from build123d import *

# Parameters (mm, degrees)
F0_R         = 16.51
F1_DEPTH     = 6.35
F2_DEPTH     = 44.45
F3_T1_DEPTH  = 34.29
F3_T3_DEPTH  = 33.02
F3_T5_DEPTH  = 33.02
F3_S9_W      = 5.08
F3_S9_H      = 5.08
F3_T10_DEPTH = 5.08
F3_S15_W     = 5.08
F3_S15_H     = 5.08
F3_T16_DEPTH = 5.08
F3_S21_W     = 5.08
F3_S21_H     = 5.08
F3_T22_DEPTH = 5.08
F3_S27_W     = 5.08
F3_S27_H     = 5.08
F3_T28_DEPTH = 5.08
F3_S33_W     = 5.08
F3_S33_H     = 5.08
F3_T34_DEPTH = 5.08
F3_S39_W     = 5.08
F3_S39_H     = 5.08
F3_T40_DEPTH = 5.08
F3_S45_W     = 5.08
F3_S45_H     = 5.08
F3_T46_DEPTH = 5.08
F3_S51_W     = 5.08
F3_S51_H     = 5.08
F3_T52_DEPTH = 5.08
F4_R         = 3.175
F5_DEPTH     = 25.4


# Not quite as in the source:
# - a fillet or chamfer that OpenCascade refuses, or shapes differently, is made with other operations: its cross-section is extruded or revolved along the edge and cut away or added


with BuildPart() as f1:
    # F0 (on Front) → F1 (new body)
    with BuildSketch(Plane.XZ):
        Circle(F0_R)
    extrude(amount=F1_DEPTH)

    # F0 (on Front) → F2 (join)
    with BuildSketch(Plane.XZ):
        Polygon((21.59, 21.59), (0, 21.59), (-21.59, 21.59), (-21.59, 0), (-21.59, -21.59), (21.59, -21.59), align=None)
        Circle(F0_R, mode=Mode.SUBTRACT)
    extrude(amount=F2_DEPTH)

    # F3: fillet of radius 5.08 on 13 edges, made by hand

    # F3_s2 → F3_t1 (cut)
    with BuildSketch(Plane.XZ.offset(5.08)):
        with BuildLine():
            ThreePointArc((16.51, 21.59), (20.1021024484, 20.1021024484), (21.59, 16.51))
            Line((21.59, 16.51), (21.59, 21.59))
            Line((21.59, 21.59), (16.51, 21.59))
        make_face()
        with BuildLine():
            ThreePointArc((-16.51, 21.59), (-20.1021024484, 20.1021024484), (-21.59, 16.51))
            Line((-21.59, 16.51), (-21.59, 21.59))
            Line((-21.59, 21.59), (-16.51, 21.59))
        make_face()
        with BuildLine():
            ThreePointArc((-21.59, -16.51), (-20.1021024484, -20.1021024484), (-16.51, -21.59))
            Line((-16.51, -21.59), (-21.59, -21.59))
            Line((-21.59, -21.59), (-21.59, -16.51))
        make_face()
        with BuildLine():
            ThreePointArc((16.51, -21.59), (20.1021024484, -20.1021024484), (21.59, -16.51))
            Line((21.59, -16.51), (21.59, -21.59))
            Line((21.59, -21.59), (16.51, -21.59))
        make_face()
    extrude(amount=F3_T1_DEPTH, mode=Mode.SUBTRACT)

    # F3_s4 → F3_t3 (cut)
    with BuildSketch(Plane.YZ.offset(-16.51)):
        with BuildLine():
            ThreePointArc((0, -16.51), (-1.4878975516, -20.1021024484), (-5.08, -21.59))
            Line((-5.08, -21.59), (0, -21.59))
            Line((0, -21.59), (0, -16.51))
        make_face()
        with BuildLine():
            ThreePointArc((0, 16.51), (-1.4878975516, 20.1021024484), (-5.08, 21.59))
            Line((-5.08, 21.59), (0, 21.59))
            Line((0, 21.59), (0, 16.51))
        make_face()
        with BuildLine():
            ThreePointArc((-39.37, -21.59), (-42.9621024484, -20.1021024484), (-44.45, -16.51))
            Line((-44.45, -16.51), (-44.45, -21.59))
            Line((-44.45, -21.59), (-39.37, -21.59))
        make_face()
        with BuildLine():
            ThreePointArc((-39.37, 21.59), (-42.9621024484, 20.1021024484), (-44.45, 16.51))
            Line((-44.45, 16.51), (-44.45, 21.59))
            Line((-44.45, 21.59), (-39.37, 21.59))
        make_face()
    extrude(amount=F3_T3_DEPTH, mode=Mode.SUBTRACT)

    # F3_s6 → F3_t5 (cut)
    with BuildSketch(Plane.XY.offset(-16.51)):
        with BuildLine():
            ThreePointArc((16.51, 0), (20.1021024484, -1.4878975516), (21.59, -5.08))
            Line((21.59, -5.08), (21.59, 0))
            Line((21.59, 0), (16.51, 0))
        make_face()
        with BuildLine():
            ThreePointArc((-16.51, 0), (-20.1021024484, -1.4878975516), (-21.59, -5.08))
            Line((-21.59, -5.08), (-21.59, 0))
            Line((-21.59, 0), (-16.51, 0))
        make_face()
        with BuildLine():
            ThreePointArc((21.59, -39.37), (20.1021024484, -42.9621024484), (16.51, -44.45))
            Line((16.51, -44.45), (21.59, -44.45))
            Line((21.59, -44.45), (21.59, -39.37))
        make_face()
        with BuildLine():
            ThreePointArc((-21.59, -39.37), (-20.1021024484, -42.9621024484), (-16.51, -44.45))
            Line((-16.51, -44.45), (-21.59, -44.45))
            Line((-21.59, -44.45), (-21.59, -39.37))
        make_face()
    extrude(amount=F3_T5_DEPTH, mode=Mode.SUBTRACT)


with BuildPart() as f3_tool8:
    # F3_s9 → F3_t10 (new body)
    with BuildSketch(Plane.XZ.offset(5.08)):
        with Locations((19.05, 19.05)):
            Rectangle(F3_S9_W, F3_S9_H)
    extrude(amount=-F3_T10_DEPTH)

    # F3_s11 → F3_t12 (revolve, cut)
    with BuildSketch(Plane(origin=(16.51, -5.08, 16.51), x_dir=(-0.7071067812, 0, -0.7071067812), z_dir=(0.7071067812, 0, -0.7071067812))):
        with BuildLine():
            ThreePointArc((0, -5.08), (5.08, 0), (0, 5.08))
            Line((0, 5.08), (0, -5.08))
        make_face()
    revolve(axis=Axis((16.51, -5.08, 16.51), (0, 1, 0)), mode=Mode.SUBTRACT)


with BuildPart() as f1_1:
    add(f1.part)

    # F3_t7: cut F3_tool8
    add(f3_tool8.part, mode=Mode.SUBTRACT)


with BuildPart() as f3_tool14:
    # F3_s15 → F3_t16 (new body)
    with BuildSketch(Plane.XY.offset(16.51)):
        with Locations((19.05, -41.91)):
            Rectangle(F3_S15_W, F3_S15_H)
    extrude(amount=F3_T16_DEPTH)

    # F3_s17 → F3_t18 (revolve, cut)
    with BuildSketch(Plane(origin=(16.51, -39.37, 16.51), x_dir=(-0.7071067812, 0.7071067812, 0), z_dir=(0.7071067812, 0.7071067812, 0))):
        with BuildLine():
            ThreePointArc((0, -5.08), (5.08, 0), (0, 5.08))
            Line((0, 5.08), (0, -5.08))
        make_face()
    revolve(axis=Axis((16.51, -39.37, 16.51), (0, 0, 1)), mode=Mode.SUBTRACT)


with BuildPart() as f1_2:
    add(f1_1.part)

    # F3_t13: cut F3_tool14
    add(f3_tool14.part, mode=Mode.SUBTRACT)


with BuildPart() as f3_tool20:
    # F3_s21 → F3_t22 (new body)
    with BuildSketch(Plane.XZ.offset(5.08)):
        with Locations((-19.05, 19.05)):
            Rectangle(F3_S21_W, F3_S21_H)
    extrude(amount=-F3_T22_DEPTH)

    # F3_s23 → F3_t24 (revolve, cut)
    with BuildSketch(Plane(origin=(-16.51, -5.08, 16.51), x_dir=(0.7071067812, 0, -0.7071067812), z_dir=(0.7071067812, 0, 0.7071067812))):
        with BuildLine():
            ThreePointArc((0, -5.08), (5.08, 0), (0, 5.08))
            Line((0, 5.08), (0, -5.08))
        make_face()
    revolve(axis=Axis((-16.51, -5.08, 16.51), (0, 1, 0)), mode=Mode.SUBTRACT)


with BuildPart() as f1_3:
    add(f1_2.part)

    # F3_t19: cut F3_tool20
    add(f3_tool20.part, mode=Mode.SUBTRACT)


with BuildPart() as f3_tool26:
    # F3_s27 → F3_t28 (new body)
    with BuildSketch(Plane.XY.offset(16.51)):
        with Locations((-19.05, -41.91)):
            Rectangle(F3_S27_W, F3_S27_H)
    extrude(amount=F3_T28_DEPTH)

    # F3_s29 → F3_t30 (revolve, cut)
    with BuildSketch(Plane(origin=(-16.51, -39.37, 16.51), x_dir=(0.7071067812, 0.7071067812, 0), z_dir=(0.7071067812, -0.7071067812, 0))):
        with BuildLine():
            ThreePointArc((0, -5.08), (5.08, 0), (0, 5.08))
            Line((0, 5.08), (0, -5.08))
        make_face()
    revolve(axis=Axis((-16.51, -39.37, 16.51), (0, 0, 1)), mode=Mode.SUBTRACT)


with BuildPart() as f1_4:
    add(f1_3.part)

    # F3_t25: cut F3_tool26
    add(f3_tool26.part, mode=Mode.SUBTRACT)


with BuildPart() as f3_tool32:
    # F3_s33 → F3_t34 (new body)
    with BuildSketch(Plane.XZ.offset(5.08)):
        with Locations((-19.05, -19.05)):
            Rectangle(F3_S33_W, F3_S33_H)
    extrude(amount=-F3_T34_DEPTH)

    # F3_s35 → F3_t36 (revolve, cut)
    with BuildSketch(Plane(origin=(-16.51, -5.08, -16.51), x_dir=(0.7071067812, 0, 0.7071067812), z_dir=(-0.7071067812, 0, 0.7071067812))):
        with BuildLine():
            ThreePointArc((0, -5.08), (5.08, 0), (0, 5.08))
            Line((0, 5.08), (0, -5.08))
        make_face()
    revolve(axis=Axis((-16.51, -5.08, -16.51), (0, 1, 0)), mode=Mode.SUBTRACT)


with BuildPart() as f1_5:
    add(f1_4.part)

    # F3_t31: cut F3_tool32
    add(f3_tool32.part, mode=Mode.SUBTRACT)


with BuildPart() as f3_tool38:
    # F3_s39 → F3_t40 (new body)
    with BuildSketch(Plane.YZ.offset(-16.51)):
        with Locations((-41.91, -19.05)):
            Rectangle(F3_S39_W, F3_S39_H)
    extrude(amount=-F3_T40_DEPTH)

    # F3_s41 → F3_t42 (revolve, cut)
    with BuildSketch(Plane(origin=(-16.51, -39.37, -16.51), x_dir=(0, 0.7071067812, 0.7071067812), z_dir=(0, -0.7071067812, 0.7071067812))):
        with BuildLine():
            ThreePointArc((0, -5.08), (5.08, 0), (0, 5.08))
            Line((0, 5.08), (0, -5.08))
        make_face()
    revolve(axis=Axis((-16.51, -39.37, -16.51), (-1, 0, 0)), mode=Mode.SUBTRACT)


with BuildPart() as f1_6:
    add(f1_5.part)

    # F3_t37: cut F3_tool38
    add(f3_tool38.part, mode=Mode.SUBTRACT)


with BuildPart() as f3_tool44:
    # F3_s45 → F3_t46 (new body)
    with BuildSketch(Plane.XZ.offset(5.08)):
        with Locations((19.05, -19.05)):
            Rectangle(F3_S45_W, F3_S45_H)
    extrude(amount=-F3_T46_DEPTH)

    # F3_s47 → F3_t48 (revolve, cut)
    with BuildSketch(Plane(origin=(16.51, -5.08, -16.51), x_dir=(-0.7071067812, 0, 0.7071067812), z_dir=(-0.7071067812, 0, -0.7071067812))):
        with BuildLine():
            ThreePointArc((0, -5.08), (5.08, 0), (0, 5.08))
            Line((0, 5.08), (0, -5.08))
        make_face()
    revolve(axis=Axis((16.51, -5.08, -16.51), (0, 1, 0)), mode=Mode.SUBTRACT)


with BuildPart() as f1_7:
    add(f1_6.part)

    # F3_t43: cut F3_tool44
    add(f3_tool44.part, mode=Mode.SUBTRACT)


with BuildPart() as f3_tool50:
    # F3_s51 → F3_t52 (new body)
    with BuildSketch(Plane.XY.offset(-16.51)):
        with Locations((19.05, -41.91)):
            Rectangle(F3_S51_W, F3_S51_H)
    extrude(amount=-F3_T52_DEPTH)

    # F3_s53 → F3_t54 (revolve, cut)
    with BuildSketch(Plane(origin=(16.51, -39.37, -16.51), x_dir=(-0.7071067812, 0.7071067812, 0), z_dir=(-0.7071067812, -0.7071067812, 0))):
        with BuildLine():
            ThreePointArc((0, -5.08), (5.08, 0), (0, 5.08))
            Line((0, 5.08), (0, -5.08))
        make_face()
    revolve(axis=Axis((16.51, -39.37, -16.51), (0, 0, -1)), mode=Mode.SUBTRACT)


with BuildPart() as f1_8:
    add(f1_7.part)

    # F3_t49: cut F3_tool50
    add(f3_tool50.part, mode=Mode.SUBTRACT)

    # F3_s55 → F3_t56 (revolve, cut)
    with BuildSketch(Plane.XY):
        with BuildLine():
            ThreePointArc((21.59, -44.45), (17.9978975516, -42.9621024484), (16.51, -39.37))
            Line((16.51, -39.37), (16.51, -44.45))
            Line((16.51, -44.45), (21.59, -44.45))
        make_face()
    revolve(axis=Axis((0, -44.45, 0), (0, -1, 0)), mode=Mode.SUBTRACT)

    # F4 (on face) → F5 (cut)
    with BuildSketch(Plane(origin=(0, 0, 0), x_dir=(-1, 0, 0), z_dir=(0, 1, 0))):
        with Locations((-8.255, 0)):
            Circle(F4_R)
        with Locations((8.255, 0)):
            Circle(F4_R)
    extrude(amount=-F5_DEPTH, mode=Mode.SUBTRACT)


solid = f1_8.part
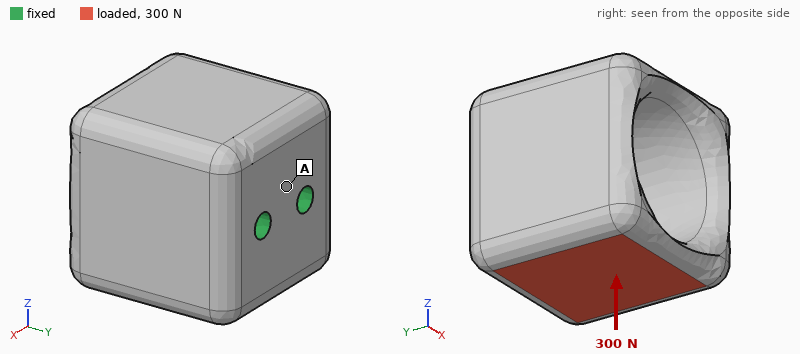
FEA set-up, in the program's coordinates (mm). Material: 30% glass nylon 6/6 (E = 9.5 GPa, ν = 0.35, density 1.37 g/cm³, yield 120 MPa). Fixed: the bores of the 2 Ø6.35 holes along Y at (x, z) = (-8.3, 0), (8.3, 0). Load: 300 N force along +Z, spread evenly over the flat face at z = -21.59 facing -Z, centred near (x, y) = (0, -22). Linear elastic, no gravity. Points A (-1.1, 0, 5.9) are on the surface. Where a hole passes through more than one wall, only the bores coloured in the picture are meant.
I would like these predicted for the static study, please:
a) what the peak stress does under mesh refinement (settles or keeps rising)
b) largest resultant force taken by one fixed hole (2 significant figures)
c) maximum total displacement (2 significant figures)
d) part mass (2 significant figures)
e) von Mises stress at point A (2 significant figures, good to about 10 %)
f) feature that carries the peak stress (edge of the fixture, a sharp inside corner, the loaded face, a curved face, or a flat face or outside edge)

keeps rising
150 N
91 µm
64 g
4.0 MPa
edge of the fixture
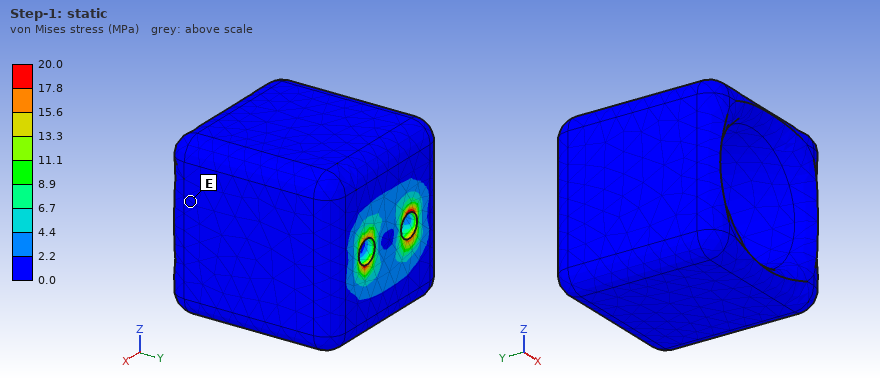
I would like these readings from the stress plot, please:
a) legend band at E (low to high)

0.0 to 2.2 MPa
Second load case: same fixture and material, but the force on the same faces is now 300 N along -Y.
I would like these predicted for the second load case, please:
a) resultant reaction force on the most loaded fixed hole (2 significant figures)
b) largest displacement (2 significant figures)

150 N
92 µm
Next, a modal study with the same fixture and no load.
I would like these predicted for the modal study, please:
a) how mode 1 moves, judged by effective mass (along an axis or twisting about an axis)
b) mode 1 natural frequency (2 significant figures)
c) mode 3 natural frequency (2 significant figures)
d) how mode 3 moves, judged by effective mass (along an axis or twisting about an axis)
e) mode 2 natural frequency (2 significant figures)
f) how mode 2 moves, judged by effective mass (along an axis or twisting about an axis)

along Z
1400 Hz
4300 Hz
twisting about Y
2200 Hz
along X
